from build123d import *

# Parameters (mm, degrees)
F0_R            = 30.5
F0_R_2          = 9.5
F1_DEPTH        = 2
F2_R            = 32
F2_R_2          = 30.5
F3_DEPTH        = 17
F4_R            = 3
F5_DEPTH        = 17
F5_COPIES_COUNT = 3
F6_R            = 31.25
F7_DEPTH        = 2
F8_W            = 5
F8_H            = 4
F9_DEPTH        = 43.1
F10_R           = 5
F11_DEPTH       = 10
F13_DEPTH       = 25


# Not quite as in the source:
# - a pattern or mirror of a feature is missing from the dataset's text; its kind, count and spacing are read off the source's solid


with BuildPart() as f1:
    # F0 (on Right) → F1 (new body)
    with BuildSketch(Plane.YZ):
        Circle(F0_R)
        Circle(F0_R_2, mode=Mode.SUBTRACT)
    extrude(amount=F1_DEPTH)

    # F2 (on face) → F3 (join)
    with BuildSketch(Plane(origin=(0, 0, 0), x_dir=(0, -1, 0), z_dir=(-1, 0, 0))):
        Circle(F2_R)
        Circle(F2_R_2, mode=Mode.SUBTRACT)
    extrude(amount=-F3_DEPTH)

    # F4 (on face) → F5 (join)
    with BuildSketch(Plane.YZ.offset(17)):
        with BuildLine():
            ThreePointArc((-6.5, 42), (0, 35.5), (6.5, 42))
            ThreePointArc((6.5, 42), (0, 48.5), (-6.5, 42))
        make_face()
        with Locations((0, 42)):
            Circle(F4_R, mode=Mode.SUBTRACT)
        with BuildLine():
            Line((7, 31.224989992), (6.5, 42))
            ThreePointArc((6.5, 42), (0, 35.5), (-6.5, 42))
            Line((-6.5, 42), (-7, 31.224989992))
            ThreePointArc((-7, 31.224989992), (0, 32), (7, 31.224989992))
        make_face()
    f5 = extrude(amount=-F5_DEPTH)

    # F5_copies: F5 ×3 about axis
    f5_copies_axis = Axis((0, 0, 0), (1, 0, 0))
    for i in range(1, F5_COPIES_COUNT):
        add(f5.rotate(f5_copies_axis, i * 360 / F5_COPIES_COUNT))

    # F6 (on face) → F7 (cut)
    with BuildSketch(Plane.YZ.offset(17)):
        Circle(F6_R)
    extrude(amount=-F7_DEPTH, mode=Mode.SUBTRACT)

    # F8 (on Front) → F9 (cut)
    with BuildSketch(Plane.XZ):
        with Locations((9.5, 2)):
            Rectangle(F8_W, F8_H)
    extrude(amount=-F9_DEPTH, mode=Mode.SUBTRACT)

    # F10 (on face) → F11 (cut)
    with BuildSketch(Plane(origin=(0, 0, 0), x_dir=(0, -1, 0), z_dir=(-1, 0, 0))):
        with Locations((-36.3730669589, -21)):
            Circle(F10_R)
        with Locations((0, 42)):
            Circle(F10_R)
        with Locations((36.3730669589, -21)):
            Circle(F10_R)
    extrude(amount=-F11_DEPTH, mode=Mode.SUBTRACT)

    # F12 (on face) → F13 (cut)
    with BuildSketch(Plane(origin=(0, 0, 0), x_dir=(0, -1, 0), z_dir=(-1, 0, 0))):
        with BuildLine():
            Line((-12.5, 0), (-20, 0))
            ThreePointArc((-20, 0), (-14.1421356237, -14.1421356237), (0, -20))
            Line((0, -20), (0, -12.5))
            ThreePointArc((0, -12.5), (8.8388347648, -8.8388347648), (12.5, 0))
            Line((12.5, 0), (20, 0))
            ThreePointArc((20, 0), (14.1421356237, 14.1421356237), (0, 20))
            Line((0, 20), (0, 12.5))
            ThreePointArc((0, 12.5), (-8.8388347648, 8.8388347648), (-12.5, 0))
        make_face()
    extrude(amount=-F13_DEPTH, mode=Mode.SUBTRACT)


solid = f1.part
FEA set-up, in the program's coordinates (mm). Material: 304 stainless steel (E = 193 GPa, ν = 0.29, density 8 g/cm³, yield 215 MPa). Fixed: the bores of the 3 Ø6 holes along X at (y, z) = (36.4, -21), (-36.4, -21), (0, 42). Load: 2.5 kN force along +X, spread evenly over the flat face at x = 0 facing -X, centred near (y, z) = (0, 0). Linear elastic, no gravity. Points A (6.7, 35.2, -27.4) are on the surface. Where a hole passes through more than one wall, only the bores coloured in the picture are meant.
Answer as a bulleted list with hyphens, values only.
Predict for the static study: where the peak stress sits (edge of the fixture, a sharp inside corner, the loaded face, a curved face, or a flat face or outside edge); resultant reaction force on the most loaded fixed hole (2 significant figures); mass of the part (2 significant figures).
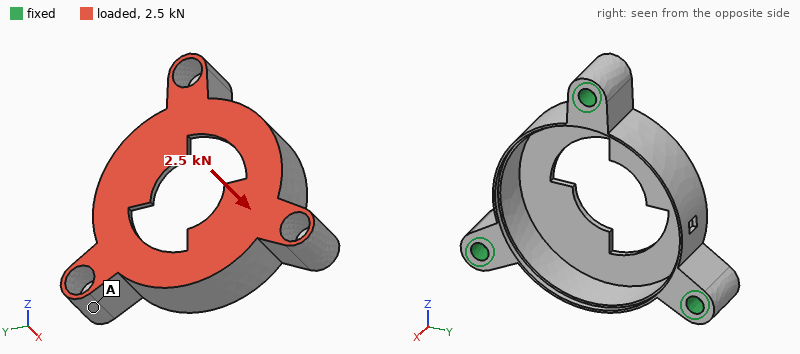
- the loaded face
- 970 N
- 130 g
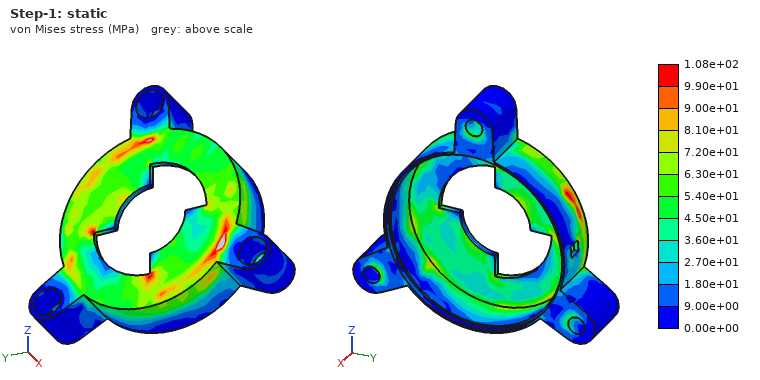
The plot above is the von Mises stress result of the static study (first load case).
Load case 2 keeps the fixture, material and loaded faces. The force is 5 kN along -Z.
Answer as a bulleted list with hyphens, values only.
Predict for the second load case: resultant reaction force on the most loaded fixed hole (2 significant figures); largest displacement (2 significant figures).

- 1.8 kN
- 34 µm
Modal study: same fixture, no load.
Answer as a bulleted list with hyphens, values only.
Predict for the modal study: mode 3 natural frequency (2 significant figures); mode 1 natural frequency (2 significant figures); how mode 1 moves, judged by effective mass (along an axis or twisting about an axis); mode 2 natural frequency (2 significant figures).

- 8900 Hz
- 6000 Hz
- along X
- 6300 Hz
